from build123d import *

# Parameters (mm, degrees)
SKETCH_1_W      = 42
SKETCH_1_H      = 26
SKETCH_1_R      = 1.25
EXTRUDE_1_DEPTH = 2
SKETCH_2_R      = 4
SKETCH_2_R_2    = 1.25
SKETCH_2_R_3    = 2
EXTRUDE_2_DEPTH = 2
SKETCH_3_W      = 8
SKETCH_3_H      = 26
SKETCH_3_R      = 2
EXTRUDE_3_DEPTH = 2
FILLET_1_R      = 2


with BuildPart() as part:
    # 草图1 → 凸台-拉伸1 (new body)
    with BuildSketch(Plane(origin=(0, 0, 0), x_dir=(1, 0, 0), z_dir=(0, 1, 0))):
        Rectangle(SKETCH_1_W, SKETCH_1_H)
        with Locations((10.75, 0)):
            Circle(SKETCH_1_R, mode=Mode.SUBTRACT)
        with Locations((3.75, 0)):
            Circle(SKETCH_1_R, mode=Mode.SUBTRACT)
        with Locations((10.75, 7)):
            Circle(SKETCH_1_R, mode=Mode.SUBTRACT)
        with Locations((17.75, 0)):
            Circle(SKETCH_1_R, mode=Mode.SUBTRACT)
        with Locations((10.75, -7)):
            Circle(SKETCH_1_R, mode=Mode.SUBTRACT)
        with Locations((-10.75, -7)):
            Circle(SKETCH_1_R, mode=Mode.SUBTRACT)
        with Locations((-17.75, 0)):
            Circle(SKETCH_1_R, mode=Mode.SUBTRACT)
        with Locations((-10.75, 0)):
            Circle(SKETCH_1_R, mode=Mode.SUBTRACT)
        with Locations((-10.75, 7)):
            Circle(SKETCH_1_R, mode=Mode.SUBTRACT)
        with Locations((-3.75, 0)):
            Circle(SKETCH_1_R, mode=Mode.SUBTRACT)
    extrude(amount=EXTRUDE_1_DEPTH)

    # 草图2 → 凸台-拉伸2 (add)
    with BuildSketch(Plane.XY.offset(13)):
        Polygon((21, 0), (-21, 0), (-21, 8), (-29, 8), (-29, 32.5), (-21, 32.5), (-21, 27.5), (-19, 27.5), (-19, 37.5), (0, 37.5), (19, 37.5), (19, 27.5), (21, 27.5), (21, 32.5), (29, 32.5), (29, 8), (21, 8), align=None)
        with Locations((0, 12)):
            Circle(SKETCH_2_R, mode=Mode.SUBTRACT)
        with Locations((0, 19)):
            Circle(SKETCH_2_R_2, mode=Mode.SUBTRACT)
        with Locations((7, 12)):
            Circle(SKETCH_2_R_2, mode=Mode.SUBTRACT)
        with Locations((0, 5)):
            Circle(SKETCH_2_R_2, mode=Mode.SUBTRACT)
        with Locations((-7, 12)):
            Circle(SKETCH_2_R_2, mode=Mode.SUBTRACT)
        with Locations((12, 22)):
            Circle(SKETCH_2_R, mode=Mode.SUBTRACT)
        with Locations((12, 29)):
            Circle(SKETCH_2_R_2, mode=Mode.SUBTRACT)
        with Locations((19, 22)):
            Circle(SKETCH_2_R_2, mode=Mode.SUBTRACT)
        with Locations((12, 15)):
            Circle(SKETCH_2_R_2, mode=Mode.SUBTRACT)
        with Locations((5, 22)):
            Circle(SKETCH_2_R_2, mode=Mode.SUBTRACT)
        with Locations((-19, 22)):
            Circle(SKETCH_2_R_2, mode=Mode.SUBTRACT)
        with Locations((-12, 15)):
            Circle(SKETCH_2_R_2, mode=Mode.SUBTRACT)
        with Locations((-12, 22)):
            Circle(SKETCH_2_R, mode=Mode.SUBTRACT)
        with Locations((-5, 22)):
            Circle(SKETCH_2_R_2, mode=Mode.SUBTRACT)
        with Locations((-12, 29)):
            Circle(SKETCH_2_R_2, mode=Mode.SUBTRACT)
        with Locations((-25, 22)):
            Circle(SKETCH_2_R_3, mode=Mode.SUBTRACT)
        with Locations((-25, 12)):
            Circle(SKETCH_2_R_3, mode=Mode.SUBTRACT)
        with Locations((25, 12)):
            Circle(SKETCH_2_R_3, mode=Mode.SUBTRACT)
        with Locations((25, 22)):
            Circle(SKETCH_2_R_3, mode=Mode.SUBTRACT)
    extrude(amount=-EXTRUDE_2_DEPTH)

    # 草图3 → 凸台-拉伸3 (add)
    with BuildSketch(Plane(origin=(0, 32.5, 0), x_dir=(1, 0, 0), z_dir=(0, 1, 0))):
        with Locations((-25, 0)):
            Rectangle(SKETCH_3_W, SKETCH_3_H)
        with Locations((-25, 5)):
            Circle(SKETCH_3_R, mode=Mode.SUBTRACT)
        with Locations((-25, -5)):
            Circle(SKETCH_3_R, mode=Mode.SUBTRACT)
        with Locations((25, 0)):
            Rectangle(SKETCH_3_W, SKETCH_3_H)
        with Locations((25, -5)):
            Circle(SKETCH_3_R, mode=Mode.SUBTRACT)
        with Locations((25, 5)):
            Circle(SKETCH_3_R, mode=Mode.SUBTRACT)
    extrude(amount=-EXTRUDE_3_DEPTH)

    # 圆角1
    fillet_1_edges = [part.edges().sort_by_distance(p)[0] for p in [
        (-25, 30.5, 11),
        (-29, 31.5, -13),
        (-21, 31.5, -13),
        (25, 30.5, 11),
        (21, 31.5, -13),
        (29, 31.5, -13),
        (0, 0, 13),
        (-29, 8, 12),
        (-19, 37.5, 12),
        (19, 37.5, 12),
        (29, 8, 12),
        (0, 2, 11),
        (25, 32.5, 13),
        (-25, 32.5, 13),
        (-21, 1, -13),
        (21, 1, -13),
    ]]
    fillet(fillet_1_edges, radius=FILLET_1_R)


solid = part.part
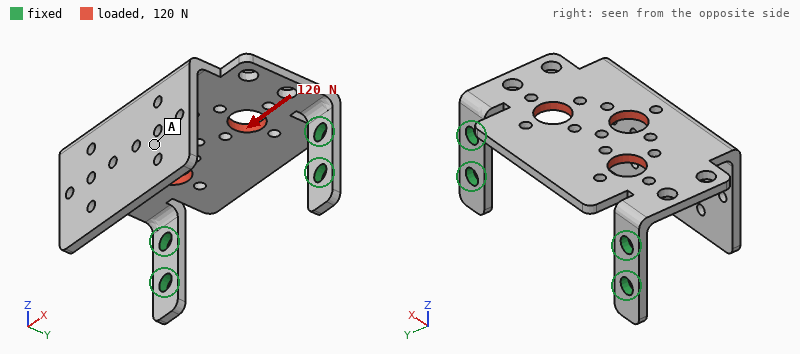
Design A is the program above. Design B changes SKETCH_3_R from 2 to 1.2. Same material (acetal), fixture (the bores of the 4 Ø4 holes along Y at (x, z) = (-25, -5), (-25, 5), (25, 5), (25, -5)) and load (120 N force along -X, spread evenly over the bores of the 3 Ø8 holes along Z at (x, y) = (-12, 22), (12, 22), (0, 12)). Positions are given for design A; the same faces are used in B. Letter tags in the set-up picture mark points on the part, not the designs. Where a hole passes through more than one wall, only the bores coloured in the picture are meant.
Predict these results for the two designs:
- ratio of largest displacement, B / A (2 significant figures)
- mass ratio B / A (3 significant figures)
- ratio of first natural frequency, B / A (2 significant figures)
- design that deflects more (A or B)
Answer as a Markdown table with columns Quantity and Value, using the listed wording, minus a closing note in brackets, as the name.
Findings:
| Quantity | Value |
|---|---|
| ratio of largest displacement, B / A | 1.4 |
| mass ratio B / A | 1.01 |
| ratio of first natural frequency, B / A | 0.96 |
| design that deflects more | B |
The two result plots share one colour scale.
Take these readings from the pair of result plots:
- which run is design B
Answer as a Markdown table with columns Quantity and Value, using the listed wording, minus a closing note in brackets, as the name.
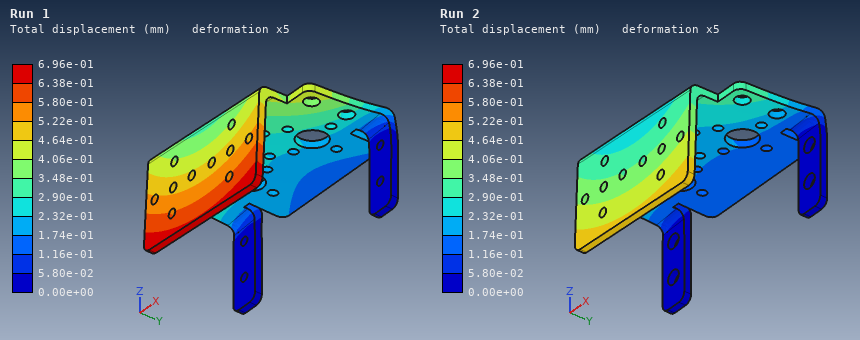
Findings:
| Quantity | Value |
|---|---|
| which run is design B | Run 1 |
